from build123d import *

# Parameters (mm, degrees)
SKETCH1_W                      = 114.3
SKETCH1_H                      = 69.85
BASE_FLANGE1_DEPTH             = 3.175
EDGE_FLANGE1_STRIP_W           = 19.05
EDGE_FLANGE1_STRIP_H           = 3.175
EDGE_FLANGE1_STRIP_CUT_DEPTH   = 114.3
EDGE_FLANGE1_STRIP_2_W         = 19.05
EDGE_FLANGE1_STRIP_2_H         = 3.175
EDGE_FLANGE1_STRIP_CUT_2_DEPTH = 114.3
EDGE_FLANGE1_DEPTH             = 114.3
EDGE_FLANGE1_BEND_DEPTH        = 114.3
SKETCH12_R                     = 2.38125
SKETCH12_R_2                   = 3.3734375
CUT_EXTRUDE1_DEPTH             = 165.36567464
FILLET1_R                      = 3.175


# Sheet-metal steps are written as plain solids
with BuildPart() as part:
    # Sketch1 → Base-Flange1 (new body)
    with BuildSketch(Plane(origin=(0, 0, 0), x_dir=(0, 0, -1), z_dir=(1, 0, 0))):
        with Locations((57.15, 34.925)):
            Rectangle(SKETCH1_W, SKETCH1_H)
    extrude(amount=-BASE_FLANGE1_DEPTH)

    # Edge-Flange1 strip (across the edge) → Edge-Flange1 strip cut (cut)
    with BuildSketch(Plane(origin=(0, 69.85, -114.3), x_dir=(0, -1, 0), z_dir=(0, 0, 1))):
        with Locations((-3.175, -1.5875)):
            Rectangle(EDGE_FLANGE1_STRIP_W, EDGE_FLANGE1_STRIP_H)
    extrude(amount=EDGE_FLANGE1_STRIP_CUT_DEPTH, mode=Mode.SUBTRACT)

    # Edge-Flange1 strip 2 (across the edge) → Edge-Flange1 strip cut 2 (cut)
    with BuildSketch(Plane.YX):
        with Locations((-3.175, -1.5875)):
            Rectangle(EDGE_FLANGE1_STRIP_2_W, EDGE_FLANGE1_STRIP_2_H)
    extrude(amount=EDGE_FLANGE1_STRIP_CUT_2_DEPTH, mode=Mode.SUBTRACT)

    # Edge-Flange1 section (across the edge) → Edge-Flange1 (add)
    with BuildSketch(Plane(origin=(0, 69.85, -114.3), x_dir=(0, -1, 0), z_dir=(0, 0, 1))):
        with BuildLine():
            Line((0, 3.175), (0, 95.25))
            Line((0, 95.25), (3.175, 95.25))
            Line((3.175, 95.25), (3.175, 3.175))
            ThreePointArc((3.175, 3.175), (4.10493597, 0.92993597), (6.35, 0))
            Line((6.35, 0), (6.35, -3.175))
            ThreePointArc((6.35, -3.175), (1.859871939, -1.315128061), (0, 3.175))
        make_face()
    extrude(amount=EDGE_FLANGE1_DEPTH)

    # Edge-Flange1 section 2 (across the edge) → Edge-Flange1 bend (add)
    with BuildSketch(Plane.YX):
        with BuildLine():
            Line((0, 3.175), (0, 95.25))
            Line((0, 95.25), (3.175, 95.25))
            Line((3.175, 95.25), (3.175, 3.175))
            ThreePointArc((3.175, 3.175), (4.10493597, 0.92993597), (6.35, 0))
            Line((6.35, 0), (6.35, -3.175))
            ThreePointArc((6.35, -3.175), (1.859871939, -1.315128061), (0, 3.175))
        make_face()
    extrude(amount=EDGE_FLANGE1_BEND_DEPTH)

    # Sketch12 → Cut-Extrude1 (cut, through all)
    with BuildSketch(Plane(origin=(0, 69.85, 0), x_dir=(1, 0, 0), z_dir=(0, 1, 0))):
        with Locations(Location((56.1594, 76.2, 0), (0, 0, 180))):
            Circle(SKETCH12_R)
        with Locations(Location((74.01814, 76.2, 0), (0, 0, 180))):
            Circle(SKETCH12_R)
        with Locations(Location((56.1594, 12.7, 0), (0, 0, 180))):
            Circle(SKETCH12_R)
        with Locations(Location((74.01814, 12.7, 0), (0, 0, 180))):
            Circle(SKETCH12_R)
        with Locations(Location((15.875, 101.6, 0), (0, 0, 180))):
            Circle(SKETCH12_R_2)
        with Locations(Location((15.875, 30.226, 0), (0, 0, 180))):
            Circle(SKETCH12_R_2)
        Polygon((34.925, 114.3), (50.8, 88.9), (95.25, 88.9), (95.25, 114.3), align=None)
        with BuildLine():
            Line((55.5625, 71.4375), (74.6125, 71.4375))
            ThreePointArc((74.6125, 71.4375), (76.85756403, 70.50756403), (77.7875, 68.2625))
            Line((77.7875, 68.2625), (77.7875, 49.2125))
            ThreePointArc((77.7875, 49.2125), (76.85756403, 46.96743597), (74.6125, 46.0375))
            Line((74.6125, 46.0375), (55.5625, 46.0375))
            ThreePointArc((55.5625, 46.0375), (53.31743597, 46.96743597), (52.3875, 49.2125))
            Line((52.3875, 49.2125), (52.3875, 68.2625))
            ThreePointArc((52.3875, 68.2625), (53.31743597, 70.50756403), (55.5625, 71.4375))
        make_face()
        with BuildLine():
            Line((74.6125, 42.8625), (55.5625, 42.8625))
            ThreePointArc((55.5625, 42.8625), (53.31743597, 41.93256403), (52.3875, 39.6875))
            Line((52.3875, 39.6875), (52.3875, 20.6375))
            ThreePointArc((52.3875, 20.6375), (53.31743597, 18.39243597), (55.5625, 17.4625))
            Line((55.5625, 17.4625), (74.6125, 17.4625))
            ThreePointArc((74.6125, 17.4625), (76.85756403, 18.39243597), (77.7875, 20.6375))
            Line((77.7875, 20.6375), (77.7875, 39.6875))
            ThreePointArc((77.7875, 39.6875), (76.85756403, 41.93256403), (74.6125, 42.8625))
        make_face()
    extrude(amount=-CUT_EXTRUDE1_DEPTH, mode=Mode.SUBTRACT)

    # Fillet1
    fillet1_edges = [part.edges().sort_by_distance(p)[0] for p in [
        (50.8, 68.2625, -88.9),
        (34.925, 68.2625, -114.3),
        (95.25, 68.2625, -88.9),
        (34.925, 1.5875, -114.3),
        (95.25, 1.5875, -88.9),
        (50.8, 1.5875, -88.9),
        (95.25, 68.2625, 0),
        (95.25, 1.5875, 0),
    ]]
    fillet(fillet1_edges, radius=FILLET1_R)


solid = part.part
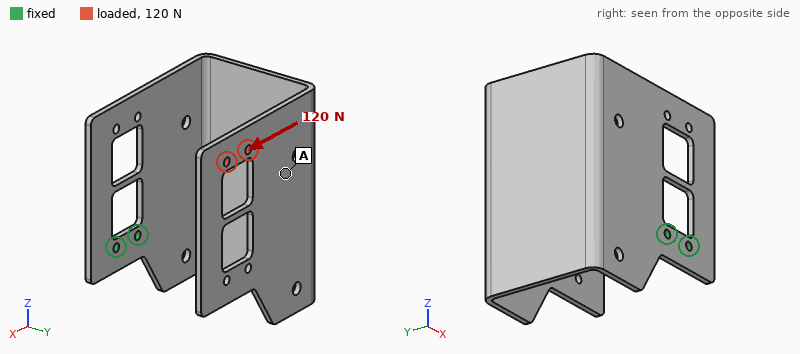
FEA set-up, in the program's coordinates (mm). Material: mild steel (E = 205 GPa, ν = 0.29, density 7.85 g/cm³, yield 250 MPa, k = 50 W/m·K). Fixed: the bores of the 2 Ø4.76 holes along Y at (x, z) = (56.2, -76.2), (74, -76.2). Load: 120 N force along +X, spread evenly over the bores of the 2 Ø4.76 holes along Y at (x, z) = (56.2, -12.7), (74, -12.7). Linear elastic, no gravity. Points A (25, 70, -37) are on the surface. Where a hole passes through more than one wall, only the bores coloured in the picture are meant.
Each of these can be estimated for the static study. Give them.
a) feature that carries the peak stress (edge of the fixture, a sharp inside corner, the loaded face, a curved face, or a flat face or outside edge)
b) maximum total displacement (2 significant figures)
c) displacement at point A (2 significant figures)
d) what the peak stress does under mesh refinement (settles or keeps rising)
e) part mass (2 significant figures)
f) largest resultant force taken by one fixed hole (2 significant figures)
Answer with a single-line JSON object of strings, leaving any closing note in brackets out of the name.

{"feature that carries the peak stress": "edge of the fixture", "maximum total displacement": "1.6 mm", "displacement at point A": "1.1 mm", "what the peak stress does under mesh refinement": "keeps rising", "part mass": "590 g", "largest resultant force taken by one fixed hole": "310 N"}
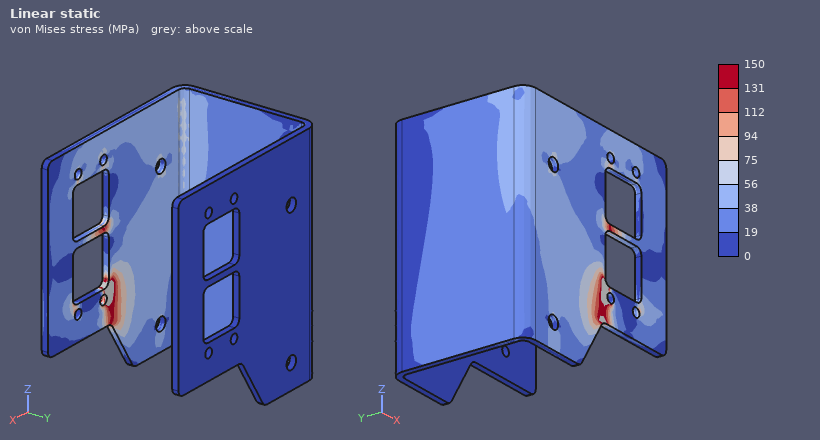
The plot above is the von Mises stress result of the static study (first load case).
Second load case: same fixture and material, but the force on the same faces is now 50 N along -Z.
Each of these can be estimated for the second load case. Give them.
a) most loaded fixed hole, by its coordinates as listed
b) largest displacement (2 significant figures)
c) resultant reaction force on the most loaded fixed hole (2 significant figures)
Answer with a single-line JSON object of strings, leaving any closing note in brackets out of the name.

{"most loaded fixed hole, by its coordinates as listed": "(56.2, -76.2)", "largest displacement": "0.56 mm", "resultant reaction force on the most loaded fixed hole": "38 N"}
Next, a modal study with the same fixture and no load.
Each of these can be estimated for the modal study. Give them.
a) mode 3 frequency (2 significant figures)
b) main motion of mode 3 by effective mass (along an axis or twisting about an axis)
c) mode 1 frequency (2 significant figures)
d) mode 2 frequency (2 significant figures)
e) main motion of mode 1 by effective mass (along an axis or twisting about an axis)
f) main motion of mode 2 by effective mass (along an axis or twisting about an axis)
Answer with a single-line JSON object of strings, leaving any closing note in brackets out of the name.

{"mode 3 frequency": "190 Hz", "main motion of mode 3 by effective mass": "along Y", "mode 1 frequency": "89 Hz", "mode 2 frequency": "100 Hz", "main motion of mode 1 by effective mass": "along X", "main motion of mode 2 by effective mass": "along Z"}
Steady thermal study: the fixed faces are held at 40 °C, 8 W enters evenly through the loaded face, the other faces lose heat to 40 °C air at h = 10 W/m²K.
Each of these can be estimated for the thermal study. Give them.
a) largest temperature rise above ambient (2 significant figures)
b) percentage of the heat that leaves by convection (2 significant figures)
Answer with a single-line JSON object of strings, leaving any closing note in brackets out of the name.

{"largest temperature rise above ambient": "71 K", "percentage of the heat that leaves by convection": "90 %"}
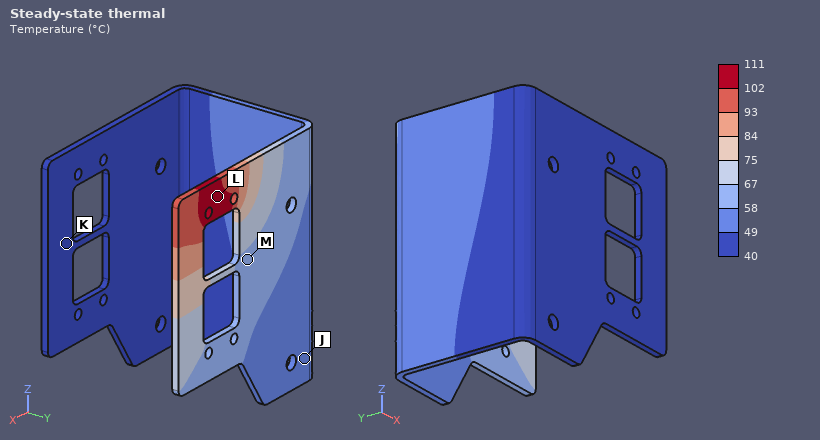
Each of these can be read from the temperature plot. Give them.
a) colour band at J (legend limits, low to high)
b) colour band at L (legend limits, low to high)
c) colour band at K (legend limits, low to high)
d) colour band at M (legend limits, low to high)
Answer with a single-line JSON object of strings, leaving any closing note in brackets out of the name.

{"colour band at J": "49 to 58 °C", "colour band at L": "102 to 111 °C", "colour band at K": "40 to 49 °C", "colour band at M": "58 to 67 °C"}
